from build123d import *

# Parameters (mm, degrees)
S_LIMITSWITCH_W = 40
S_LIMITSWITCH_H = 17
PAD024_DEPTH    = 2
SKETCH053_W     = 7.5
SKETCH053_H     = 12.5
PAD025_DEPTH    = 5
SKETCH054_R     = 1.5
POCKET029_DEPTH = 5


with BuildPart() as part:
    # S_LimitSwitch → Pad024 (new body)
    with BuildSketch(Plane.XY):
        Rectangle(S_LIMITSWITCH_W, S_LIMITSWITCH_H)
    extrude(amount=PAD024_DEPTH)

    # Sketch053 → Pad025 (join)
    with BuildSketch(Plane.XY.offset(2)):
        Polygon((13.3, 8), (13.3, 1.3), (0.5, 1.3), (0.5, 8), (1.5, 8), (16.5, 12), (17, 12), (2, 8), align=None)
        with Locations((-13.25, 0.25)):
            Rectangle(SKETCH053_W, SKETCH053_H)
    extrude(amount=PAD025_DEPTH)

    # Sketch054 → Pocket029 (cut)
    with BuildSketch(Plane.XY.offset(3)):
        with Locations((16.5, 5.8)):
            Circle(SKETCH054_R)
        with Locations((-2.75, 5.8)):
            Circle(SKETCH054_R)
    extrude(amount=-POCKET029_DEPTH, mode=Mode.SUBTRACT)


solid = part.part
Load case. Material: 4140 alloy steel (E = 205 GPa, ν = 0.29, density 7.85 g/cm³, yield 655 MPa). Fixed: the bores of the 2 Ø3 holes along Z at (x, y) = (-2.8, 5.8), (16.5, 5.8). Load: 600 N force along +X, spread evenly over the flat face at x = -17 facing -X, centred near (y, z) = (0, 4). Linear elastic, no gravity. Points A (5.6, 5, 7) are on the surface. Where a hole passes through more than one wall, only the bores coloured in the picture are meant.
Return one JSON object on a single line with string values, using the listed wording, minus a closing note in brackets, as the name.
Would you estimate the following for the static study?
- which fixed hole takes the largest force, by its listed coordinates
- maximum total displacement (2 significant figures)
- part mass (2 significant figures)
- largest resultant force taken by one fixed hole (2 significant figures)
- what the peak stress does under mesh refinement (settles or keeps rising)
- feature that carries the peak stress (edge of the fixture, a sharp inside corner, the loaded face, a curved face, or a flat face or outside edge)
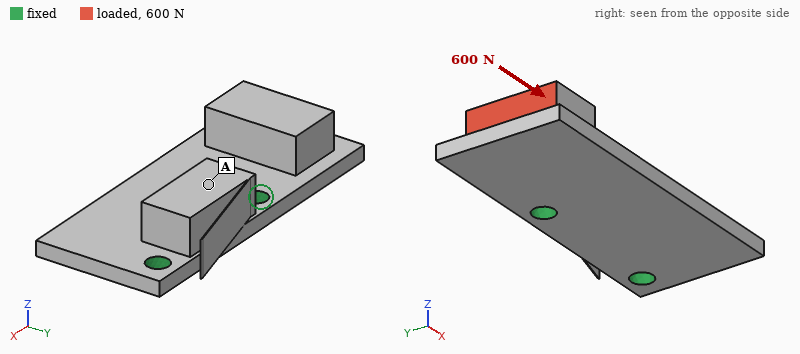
{"which fixed hole takes the largest force, by its listed coordinates": "(-2.8, 5.8)", "maximum total displacement": "0.11 mm", "part mass": "18 g", "largest resultant force taken by one fixed hole": "440 N", "what the peak stress does under mesh refinement": "keeps rising", "feature that carries the peak stress": "edge of the fixture"}
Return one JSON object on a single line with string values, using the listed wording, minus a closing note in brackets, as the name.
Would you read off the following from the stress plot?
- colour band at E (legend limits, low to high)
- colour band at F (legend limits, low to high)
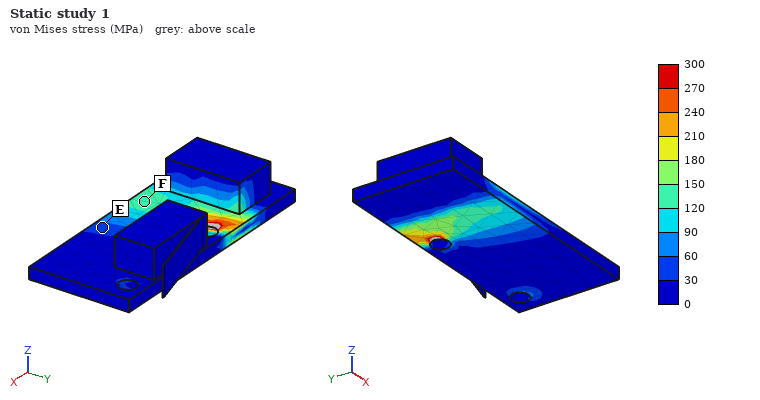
{"colour band at E": "30 to 60 MPa", "colour band at F": "120 to 150 MPa"}
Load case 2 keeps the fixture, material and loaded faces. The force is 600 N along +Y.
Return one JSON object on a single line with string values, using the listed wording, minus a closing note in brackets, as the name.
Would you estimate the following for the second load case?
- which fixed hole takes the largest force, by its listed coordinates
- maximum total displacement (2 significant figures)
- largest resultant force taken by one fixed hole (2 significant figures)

{"which fixed hole takes the largest force, by its listed coordinates": "(-2.8, 5.8)", "maximum total displacement": "69 µm", "largest resultant force taken by one fixed hole": "1.0 kN"}
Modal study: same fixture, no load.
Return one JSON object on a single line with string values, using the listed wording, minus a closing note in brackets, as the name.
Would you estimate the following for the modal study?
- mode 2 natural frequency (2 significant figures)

{"mode 2 natural frequency": "3300 Hz"}
